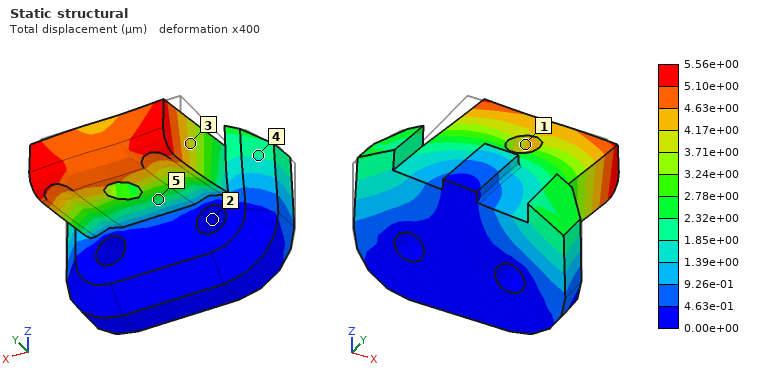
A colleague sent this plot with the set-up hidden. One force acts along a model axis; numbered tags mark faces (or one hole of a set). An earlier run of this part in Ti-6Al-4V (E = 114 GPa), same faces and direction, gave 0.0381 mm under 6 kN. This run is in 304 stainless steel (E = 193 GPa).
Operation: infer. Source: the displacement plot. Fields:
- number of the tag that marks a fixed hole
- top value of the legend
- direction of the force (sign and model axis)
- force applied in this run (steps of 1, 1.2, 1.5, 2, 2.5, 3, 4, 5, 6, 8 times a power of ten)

2
5.56e+00 µm
+X
1.5 kN
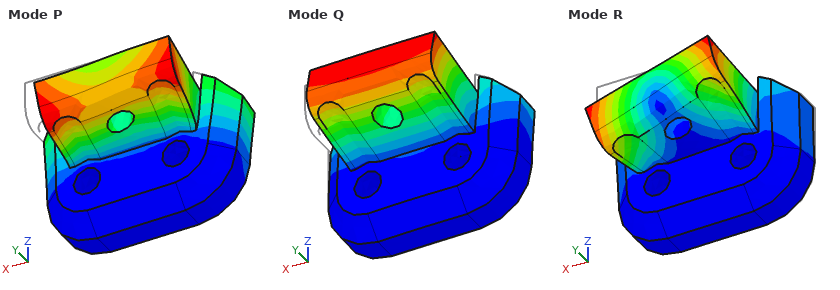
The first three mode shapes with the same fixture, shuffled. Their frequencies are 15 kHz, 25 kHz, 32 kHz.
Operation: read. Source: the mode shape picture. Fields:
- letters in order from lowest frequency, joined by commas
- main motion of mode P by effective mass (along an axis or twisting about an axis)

Q, P, R
along X
